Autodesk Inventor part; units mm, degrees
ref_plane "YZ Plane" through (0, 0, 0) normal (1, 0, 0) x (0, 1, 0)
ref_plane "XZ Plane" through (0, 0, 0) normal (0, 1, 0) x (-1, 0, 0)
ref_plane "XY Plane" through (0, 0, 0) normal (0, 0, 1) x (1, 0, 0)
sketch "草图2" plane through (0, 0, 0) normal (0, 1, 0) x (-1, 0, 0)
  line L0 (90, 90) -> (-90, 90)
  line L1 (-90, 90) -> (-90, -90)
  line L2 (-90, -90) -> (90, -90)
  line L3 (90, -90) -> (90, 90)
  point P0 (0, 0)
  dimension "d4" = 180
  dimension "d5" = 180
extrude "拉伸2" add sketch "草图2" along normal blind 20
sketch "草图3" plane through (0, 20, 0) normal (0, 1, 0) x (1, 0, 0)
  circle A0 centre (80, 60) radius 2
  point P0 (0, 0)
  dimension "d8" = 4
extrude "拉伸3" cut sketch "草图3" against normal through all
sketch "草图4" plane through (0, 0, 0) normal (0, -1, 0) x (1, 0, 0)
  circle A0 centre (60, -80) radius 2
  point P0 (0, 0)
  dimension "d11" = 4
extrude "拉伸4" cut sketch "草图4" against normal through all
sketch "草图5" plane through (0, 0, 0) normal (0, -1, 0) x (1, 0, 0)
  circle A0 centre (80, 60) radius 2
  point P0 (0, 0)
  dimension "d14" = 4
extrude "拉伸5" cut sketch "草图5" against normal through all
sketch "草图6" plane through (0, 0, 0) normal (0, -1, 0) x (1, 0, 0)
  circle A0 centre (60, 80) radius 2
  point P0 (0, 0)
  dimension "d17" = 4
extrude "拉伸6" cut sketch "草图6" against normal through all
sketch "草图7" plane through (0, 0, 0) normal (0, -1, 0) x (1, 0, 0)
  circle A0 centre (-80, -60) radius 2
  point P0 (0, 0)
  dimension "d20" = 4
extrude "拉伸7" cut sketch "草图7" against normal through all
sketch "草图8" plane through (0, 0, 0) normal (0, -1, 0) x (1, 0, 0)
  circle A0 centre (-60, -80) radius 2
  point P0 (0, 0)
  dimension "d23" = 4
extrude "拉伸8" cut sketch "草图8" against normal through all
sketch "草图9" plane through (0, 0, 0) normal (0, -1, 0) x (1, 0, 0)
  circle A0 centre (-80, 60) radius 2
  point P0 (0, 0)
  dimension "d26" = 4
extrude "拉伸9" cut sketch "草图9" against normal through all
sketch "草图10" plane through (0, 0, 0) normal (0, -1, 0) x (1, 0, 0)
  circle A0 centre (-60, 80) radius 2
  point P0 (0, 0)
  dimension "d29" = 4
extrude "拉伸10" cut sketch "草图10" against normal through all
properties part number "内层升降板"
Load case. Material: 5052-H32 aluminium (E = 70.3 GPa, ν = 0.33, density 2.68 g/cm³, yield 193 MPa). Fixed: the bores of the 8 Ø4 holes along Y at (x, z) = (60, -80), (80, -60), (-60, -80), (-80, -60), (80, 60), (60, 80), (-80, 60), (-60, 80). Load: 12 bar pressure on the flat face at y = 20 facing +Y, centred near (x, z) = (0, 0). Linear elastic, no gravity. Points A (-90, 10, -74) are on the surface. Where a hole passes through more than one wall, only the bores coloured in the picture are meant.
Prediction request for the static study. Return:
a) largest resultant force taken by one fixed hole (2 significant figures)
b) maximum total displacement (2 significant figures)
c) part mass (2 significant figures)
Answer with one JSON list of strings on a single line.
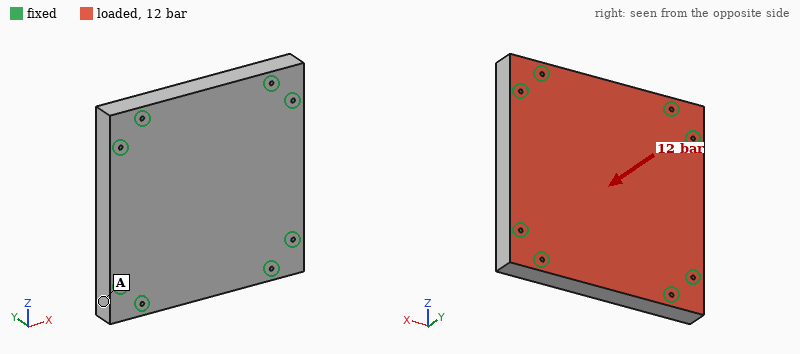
["4.9 kN", "83 µm", "1.7 kg"]
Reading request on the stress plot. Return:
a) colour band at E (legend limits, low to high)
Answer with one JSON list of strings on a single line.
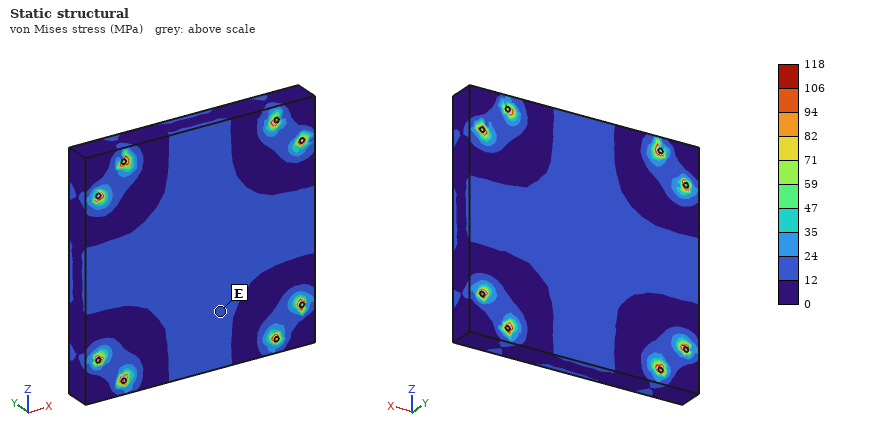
["12 to 24 MPa"]
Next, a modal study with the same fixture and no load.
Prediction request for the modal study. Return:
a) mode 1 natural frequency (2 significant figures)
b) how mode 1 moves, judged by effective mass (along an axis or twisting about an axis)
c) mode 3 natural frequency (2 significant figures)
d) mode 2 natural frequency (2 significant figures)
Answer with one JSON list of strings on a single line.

["3200 Hz", "along Y", "5500 Hz", "5500 Hz"]
